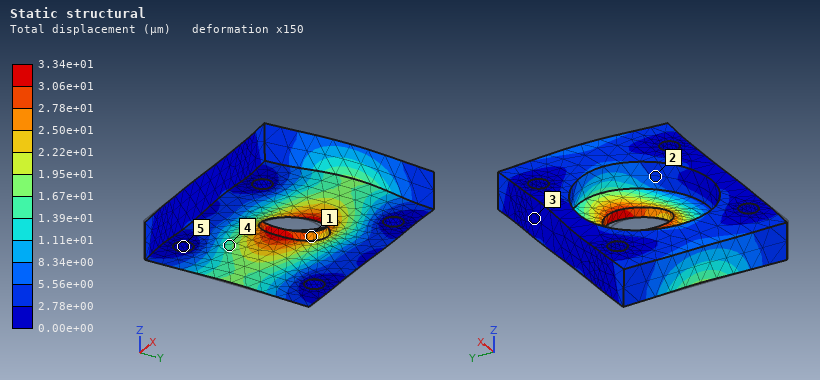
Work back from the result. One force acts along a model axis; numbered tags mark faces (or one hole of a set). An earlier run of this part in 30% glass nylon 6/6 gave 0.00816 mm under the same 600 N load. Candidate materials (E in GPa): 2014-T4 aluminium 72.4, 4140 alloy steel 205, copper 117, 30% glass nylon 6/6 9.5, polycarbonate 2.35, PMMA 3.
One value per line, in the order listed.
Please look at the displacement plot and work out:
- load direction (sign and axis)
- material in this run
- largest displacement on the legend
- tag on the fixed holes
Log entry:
+X
polycarbonate
3.34e+01 µm
5
